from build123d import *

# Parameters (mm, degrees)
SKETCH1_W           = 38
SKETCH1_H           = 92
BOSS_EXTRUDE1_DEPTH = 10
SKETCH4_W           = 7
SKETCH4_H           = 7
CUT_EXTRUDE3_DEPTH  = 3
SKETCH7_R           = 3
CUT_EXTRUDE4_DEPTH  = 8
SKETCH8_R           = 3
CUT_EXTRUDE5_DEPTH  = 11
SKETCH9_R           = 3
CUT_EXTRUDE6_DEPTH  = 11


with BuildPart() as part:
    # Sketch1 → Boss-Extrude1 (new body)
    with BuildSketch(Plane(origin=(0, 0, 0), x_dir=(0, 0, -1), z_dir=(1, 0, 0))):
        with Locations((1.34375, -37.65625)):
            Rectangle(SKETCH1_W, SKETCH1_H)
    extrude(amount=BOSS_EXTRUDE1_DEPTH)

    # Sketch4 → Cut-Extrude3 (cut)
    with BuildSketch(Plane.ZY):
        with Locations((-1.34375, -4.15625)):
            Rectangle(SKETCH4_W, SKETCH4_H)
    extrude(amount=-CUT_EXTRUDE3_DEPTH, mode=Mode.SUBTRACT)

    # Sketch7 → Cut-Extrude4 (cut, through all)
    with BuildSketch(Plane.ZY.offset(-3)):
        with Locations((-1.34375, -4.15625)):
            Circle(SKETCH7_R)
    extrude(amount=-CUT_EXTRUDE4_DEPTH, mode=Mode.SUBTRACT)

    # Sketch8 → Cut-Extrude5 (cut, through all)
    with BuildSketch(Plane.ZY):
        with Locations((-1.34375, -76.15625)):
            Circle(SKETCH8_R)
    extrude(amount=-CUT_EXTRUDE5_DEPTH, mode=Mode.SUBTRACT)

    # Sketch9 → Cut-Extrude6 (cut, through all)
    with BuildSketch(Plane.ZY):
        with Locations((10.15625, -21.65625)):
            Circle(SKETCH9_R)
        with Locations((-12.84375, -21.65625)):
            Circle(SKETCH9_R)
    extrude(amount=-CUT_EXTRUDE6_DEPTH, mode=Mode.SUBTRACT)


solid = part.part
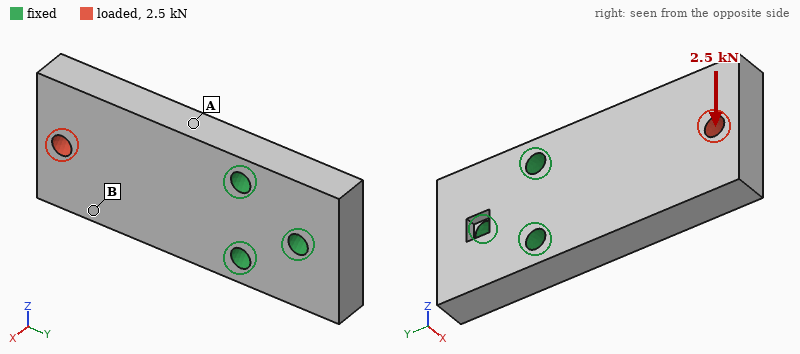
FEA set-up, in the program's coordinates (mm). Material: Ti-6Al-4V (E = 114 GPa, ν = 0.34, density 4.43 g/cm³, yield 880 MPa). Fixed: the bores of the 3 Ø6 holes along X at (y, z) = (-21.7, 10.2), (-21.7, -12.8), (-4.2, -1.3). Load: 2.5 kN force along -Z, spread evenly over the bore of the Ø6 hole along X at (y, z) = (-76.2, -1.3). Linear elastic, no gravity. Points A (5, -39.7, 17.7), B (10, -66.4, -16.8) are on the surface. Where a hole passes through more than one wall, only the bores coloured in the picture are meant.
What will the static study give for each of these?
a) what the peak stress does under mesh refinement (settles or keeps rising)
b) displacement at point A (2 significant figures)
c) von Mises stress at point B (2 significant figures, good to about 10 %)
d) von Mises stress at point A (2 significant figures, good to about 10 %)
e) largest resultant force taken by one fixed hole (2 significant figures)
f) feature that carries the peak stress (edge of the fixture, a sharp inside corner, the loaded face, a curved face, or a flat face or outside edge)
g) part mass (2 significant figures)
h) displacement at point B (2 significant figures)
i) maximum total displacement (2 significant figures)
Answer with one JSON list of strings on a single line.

["keeps rising", "11 µm", "10 MPa", "37 MPa", "5.1 kN", "edge of the fixture", "150 g", "29 µm", "44 µm"]
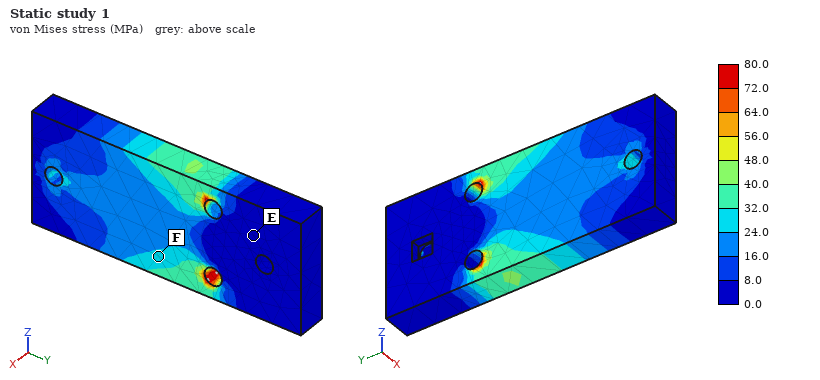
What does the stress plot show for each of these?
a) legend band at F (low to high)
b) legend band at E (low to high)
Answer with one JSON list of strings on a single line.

["24.0 to 32.0 MPa", "0.0 to 8.0 MPa"]
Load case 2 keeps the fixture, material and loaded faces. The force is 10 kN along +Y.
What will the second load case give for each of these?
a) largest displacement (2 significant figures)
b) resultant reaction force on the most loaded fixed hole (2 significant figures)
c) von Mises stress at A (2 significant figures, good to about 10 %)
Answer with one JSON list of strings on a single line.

["21 µm", "4.7 kN", "25 MPa"]
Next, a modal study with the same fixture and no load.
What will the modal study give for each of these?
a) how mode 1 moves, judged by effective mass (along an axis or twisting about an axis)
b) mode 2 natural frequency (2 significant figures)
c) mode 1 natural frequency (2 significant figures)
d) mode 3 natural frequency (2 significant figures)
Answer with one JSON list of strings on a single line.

["along X", "6500 Hz", "2200 Hz", "6700 Hz"]
